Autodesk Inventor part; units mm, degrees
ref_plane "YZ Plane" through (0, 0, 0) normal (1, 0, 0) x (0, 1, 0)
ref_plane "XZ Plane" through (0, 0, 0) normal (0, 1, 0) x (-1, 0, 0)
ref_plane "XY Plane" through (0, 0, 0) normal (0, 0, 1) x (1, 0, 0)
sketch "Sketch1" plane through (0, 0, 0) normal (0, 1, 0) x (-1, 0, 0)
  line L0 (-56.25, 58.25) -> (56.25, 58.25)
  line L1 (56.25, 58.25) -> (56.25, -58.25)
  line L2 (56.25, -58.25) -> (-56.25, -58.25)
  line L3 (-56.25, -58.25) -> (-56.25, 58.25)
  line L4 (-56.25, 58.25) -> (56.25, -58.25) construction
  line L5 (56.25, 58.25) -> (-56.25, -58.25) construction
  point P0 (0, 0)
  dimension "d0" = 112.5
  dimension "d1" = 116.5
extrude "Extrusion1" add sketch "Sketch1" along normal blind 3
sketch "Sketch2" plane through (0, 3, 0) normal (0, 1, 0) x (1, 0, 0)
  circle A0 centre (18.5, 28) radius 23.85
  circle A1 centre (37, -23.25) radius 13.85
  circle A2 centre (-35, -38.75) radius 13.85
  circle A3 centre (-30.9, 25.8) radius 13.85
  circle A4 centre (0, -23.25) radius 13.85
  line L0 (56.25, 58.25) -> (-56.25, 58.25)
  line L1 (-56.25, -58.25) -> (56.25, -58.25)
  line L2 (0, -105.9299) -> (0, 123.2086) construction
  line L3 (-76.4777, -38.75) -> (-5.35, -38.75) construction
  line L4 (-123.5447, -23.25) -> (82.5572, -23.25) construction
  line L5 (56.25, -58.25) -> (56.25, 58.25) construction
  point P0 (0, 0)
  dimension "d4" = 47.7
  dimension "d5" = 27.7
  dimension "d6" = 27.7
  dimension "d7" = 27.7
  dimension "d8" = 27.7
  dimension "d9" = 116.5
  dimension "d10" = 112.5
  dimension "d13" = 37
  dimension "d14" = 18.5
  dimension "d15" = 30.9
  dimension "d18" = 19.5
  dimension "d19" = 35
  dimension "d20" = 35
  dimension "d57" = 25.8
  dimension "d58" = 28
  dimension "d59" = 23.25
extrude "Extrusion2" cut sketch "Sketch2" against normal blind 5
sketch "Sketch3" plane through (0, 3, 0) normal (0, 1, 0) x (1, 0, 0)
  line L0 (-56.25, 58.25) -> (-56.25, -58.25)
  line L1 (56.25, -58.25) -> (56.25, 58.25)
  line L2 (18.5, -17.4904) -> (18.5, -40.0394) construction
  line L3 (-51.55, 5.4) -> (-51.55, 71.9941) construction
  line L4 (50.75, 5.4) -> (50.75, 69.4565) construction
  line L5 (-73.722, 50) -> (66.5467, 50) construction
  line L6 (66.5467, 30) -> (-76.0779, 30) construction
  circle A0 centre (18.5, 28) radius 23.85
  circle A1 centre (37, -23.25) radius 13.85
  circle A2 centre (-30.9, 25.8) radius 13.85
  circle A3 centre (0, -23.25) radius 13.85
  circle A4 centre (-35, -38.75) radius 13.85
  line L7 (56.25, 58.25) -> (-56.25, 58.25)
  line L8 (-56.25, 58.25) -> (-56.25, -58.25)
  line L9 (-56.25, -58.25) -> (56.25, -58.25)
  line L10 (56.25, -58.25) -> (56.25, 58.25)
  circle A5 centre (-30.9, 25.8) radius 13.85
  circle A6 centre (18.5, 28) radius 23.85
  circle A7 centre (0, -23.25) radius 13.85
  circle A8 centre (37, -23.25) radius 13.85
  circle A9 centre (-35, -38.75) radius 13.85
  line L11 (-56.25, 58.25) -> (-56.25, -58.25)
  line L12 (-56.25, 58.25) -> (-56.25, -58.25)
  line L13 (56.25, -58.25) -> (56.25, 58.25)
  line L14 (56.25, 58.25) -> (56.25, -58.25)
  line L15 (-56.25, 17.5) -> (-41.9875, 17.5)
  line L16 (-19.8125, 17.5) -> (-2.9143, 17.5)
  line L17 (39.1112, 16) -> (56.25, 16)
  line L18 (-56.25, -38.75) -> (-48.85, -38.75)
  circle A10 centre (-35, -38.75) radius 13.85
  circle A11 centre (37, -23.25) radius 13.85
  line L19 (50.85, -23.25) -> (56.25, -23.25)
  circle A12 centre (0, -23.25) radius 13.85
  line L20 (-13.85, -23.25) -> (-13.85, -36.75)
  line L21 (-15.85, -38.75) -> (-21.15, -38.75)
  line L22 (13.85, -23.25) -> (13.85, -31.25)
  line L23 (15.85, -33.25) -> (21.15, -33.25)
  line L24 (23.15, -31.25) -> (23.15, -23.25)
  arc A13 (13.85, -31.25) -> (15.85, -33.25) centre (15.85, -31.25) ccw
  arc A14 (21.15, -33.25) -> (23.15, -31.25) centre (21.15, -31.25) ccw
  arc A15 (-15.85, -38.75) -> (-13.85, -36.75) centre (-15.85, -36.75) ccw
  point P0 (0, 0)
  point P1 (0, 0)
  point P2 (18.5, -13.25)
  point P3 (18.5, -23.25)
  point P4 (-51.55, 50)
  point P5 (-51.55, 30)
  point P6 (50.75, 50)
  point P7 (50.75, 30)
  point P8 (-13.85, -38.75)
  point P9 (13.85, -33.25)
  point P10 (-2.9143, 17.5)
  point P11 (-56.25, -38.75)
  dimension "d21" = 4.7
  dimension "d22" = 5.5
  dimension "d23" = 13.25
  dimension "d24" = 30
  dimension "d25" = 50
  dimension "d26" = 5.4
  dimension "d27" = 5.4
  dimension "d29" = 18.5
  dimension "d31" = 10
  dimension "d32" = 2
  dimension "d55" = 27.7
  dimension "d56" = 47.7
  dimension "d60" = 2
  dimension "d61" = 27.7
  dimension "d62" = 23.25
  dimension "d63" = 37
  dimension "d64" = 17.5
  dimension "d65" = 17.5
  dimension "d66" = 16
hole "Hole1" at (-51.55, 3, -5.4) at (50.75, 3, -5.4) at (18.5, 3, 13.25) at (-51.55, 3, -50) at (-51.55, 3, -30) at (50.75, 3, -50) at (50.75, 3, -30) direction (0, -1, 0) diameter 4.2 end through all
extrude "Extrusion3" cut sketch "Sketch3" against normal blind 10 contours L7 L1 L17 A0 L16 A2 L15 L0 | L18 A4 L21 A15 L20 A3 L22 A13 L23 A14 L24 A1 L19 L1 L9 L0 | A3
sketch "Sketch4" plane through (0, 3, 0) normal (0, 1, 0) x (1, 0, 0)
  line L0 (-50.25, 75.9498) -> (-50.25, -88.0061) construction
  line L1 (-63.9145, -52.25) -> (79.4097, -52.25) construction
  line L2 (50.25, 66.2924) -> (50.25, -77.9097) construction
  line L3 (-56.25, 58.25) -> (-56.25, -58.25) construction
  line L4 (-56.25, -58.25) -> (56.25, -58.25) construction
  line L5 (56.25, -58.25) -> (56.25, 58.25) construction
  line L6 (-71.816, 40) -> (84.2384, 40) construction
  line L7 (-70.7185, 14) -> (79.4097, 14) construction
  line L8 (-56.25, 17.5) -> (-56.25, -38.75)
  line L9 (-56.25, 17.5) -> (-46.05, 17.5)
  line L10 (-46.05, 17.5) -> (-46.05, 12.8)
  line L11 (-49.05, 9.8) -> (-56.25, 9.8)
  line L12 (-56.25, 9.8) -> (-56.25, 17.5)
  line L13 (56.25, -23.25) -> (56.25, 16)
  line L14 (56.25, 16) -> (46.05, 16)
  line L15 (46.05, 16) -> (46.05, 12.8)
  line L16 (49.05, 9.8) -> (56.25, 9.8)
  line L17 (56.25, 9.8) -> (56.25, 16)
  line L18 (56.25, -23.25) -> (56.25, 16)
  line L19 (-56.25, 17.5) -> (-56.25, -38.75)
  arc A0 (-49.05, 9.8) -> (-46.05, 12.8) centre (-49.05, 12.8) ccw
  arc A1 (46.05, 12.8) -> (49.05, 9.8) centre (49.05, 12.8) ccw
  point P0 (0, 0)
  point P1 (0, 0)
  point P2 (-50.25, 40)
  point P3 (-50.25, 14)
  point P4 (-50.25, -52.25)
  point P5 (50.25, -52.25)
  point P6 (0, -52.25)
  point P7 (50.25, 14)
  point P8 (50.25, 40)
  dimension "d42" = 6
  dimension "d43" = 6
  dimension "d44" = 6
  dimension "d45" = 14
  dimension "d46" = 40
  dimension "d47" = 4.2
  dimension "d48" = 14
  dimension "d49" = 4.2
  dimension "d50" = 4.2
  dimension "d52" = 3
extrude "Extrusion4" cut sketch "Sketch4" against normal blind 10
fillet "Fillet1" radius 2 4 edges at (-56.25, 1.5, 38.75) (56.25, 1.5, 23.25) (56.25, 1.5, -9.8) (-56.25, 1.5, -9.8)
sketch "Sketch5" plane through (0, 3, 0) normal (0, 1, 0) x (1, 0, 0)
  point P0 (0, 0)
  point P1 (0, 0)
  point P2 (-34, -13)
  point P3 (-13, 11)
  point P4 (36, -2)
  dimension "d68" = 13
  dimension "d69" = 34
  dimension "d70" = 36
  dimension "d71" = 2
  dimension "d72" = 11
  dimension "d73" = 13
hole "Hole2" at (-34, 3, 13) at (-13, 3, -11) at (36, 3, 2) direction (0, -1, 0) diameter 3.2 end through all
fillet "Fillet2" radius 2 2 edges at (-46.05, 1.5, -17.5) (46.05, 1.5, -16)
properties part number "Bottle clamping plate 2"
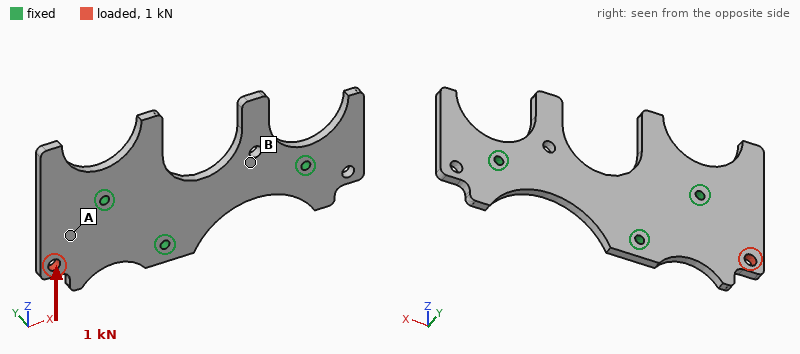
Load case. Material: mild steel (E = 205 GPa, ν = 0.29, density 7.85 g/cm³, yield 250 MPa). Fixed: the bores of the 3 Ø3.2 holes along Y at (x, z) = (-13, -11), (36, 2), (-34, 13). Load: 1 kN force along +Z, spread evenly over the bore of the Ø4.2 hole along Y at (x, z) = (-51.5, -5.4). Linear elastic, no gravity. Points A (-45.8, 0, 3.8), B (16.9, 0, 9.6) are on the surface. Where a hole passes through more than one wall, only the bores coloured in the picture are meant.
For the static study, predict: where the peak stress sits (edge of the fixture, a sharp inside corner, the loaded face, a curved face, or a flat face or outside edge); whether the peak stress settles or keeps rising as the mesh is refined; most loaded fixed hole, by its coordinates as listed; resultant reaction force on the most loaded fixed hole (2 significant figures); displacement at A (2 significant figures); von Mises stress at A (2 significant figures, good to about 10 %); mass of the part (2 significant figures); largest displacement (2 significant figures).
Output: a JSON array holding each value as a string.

["edge of the fixture", "keeps rising", "(-34, 13)", "1.3 kN", "3.8 µm", "23 MPa", "87 g", "8.3 µm"]
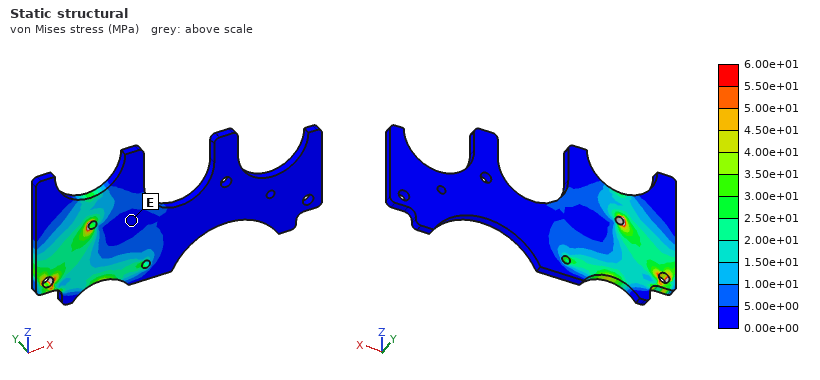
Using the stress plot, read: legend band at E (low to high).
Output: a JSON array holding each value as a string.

["0.00e+00 to 5.00e+00 MPa"]
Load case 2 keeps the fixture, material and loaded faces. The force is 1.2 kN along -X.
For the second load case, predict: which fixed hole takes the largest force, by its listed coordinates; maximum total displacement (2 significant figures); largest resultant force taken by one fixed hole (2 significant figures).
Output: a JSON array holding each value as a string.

["(-13, -11)", "7.2 µm", "750 N"]
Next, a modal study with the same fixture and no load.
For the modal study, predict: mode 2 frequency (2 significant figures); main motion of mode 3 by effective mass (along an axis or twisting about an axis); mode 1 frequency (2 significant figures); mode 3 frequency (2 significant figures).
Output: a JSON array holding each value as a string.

["3300 Hz", "twisting about X", "2600 Hz", "3400 Hz"]
